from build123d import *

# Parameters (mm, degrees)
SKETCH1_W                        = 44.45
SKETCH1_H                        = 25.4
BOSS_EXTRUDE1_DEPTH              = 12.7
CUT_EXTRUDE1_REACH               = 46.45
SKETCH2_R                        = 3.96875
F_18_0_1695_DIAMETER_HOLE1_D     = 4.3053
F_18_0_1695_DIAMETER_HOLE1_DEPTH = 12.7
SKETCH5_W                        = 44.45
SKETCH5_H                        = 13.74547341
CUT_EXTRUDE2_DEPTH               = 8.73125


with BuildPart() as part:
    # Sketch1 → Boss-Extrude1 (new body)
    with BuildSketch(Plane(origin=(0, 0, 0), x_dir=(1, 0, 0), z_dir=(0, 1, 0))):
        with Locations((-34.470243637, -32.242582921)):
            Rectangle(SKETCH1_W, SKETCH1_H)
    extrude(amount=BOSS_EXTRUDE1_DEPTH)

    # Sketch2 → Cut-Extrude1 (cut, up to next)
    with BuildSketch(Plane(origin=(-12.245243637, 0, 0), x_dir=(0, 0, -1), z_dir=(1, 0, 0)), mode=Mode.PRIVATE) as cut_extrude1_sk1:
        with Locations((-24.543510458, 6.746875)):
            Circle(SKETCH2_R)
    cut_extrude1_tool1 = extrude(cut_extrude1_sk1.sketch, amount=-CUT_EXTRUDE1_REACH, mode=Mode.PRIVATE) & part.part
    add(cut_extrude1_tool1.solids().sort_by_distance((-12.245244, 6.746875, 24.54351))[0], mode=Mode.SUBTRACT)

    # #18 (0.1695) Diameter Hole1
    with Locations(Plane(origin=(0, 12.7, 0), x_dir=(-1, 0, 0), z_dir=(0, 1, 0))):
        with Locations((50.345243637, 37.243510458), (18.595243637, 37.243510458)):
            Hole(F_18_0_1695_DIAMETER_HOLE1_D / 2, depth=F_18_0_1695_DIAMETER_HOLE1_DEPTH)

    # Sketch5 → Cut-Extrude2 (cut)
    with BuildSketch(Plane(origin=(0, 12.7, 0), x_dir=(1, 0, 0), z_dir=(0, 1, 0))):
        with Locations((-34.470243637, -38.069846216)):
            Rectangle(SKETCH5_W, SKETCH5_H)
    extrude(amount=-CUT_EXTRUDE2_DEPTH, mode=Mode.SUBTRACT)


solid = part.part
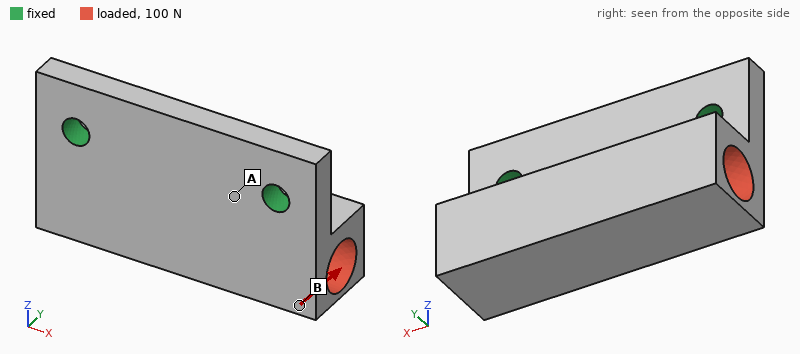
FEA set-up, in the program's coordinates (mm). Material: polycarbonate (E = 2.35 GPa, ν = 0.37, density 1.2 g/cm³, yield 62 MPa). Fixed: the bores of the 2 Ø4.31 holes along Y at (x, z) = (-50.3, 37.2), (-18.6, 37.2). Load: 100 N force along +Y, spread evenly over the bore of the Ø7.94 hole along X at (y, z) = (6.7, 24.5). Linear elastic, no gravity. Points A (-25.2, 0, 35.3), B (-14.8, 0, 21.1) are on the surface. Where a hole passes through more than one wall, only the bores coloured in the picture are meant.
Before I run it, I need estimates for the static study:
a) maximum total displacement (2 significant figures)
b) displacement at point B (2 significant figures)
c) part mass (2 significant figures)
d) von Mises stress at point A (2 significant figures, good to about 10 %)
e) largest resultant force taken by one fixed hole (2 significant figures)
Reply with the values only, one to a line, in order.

0.27 mm
0.19 mm
8.0 g
4.6 MPa
50 N
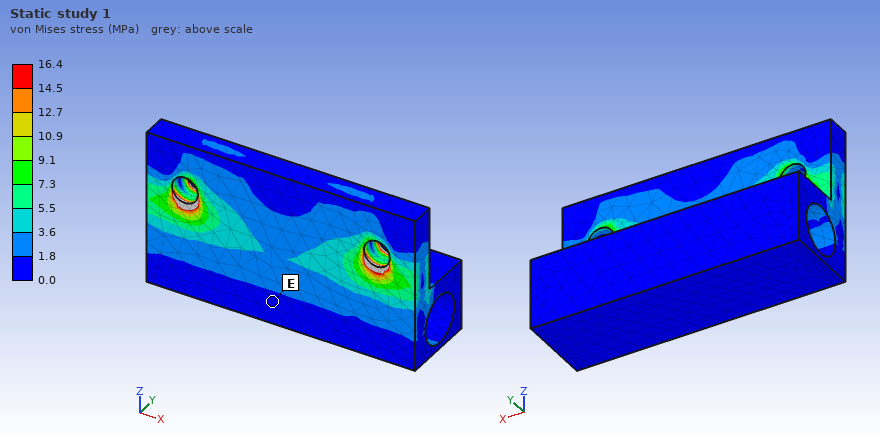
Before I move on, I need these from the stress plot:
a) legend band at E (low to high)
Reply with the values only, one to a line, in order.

0.0 to 1.8 MPa
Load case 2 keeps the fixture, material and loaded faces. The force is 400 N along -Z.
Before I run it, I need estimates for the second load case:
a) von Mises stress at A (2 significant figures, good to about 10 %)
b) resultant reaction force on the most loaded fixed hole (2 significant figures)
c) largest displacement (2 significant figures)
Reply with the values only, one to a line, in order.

8.2 MPa
200 N
0.58 mm
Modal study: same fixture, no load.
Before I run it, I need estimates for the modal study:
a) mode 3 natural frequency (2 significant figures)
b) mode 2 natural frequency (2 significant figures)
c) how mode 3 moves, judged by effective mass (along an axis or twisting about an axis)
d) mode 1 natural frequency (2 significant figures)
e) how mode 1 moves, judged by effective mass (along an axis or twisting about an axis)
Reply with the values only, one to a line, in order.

5600 Hz
4200 Hz
along Y
1600 Hz
along Y
